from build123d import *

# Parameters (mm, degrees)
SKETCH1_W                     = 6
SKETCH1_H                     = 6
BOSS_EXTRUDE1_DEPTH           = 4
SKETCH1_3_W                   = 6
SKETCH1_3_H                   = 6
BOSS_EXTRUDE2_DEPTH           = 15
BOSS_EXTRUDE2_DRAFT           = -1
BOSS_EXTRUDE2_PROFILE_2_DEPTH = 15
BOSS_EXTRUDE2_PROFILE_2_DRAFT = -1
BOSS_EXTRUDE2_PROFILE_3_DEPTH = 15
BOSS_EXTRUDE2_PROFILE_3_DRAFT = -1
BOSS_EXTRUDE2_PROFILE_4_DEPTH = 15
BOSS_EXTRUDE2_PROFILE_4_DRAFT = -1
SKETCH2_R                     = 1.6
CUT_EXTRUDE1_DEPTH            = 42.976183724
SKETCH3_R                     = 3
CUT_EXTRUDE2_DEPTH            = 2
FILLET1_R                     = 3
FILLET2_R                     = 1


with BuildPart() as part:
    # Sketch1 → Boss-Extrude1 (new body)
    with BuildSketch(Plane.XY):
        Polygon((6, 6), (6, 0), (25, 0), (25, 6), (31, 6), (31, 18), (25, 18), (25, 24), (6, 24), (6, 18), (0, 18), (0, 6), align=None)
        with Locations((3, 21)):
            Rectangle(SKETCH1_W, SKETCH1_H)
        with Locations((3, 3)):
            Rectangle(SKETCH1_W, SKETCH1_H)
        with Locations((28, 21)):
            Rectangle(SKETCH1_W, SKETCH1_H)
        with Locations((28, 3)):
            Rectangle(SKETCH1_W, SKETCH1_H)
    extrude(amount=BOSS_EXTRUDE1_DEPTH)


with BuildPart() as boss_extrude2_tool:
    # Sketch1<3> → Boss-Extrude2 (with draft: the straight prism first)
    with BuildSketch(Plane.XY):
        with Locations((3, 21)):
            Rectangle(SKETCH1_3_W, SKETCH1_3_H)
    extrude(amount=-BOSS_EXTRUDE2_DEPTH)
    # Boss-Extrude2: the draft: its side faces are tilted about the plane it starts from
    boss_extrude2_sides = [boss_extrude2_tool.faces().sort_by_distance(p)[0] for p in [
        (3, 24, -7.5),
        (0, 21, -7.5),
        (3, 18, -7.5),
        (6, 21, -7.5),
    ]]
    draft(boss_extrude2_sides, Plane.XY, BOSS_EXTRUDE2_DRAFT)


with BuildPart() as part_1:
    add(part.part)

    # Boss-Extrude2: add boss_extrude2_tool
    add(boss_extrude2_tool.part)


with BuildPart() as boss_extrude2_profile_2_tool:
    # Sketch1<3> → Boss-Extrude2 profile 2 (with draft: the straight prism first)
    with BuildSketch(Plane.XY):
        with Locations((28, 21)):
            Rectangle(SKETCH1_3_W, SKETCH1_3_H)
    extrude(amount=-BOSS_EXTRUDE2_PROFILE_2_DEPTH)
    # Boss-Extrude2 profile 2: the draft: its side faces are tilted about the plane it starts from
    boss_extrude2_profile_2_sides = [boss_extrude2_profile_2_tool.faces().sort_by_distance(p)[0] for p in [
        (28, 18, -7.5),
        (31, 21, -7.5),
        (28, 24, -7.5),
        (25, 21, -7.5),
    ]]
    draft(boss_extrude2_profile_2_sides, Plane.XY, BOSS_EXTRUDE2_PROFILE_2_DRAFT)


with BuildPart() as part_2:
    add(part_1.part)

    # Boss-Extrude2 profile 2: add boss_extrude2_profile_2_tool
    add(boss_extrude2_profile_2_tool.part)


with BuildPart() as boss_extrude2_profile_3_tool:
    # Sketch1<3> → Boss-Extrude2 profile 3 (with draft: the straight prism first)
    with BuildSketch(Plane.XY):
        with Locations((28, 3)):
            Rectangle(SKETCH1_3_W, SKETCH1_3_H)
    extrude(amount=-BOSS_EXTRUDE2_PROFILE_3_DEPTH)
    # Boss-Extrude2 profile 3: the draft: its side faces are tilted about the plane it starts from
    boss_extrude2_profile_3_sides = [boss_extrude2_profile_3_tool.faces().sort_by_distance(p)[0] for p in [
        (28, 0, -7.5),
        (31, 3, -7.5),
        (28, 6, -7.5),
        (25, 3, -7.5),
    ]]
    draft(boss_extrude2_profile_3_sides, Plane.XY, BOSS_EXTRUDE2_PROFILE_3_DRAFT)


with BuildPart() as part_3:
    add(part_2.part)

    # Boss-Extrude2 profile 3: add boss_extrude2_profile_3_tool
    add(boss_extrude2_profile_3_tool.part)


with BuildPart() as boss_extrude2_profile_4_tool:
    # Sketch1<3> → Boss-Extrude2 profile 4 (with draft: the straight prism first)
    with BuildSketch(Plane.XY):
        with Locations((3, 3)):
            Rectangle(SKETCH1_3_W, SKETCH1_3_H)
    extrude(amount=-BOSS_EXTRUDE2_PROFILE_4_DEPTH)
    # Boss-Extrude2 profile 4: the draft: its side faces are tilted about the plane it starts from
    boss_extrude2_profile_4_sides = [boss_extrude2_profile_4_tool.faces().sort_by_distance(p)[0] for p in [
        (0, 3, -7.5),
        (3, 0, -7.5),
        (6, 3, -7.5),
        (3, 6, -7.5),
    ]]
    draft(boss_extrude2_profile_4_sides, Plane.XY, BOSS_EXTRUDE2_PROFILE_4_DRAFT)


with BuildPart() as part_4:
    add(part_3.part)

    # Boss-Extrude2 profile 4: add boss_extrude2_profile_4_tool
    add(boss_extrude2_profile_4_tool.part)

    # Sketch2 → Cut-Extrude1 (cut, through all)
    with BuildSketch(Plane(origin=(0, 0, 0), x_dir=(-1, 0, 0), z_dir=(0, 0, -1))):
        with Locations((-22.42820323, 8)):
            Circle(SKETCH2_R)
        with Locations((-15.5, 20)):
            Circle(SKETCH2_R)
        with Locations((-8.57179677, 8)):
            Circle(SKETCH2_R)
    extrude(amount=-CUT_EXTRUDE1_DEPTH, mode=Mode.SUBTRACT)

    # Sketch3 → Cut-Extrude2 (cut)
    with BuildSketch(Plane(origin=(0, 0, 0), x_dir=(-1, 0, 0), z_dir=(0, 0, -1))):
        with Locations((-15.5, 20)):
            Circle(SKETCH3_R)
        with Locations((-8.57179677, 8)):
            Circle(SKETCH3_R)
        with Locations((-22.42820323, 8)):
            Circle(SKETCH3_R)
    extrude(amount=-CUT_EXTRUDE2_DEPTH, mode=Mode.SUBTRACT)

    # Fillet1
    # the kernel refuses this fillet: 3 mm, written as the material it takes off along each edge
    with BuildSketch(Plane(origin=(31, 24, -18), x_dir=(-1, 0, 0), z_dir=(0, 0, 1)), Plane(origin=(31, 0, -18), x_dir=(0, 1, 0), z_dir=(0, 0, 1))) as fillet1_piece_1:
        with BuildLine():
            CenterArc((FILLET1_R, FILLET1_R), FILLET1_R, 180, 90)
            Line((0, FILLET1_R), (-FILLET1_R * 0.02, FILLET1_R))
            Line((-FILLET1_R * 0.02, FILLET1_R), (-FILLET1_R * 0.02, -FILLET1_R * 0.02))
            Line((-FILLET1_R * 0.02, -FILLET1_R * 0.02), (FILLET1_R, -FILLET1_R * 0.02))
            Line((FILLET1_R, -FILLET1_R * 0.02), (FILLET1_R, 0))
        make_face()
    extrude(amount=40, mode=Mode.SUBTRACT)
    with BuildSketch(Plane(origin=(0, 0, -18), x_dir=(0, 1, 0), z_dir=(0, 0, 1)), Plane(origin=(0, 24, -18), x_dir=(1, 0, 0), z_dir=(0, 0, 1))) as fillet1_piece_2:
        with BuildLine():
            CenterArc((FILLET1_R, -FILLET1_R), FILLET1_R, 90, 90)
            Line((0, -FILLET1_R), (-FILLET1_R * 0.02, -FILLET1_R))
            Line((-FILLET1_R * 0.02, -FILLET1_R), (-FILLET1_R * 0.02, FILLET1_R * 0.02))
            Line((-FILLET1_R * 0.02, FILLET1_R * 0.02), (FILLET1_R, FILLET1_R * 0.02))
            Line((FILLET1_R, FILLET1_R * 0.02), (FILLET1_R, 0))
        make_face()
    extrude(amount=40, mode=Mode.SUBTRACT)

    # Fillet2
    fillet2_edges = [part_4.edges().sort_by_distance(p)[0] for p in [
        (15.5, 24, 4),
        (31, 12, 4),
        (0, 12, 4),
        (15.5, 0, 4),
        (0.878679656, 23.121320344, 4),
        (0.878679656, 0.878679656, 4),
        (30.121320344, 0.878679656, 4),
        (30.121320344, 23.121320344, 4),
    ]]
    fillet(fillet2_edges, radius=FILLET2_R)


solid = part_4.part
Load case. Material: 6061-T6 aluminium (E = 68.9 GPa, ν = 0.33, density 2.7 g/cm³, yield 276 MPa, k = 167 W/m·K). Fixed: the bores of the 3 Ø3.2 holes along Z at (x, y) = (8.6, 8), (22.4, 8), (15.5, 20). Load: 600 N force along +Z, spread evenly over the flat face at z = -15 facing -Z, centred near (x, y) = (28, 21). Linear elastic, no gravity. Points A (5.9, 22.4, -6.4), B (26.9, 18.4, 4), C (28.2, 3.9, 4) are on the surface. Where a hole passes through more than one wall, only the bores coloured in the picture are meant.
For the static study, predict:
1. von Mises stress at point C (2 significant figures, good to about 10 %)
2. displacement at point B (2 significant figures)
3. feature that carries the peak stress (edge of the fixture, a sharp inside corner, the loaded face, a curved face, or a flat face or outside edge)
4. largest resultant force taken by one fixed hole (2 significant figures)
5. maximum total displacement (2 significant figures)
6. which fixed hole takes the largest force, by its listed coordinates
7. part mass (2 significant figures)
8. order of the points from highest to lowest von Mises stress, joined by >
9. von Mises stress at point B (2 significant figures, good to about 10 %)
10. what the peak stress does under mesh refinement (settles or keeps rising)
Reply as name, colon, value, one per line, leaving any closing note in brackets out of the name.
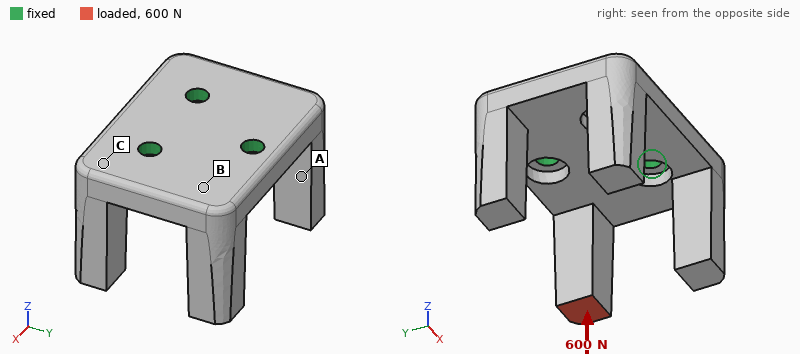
von Mises stress at point C: 30 MPa
displacement at point B: 0.056 mm
feature that carries the peak stress: edge of the fixture
largest resultant force taken by one fixed hole: 570 N
maximum total displacement: 0.19 mm
which fixed hole takes the largest force, by its listed coordinates: (15.5, 20)
part mass: 12 g
order of the points from highest to lowest von Mises stress, joined by >: B > C > A
von Mises stress at point B: 59 MPa
what the peak stress does under mesh refinement: keeps rising
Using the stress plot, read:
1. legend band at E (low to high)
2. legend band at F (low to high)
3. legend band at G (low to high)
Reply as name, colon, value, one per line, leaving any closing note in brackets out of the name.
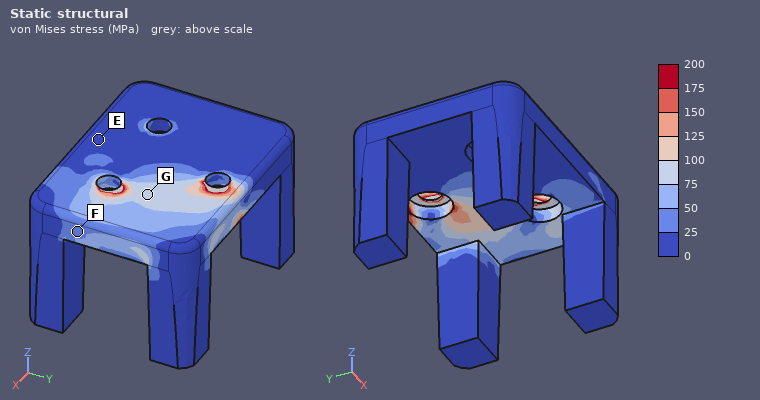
legend band at E: 0 to 25 MPa
legend band at F: 25 to 50 MPa
legend band at G: 75 to 100 MPa
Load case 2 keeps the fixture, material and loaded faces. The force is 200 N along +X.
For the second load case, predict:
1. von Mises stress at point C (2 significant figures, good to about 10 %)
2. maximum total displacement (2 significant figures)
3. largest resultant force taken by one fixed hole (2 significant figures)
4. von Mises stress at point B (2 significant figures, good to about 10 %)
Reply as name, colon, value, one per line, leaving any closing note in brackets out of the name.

von Mises stress at point C: 20 MPa
maximum total displacement: 0.18 mm
largest resultant force taken by one fixed hole: 270 N
von Mises stress at point B: 75 MPa
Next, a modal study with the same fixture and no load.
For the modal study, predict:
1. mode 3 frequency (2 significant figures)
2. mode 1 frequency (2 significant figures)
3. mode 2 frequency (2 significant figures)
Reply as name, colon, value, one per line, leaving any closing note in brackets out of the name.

mode 3 frequency: 7500 Hz
mode 1 frequency: 6300 Hz
mode 2 frequency: 6500 Hz
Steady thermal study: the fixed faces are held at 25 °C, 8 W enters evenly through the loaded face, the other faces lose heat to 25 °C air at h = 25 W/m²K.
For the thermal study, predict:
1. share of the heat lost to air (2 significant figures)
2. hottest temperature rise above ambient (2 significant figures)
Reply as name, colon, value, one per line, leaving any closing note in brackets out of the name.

share of the heat lost to air: 3.4 %
hottest temperature rise above ambient: 33 K
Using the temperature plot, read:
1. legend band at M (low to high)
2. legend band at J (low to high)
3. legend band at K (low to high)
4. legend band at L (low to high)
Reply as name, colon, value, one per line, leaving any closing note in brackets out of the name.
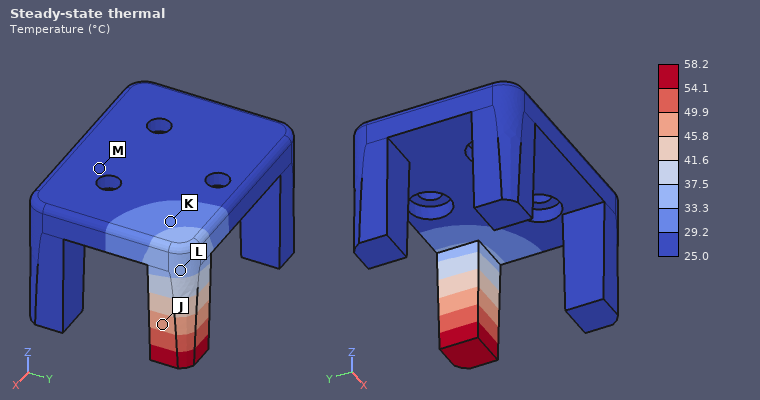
legend band at M: 25.0 to 29.2 °C
legend band at J: 45.8 to 49.9 °C
legend band at K: 29.2 to 33.3 °C
legend band at L: 33.3 to 37.5 °C
